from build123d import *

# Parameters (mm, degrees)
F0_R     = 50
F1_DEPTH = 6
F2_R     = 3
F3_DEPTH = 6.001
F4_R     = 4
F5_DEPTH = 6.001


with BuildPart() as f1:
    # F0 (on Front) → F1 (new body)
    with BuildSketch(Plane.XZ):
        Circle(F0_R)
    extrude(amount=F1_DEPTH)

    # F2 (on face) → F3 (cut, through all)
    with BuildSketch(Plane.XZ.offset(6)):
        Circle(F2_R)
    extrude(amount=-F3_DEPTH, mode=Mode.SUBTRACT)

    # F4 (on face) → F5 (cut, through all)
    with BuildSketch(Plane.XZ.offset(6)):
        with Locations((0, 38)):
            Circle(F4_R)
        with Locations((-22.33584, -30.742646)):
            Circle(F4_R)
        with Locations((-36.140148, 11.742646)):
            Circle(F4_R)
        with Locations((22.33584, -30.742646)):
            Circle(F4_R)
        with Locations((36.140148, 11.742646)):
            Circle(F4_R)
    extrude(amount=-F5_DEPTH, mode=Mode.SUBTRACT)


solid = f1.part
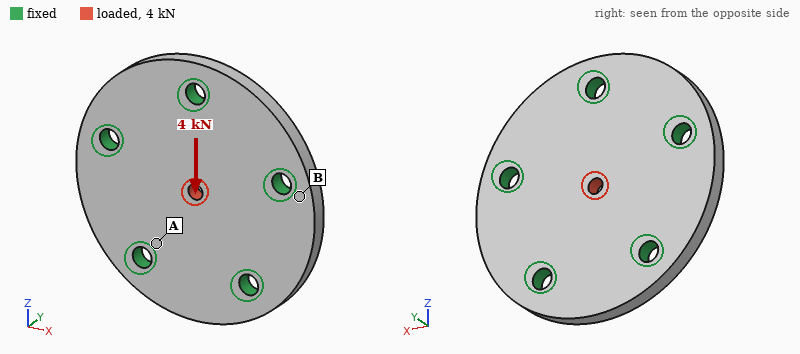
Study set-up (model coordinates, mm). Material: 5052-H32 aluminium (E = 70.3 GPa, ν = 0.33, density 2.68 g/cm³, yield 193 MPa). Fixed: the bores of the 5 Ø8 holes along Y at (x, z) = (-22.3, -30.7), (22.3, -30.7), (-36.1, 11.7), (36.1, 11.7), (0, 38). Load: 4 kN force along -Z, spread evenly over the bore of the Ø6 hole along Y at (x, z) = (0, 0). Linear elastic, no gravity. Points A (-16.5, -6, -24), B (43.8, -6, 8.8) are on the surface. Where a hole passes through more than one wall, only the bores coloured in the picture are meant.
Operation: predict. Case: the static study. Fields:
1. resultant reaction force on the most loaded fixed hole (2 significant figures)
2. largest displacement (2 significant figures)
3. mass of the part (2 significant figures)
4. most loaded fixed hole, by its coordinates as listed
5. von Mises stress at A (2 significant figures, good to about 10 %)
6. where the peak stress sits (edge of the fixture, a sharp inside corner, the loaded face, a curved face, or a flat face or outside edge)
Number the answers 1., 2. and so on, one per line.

1. 1.2 kN
2. 7.2 µm
3. 120 g
4. (0, 38)
5. 11 MPa
6. the loaded face
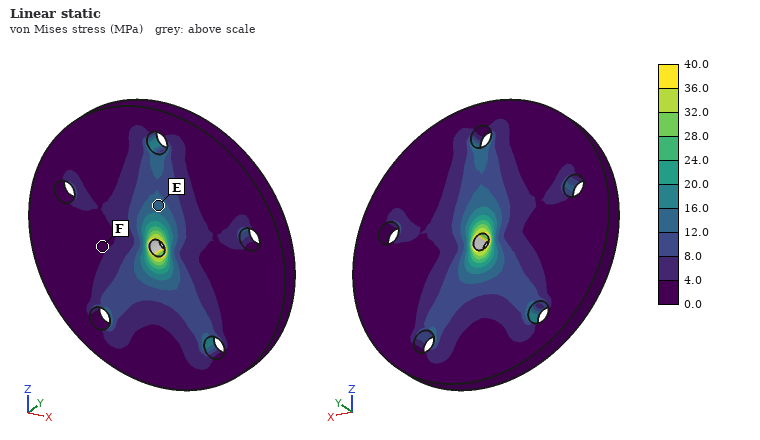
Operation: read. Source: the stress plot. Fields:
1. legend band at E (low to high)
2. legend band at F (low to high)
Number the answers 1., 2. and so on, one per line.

1. 12.0 to 16.0 MPa
2. 0.0 to 4.0 MPa
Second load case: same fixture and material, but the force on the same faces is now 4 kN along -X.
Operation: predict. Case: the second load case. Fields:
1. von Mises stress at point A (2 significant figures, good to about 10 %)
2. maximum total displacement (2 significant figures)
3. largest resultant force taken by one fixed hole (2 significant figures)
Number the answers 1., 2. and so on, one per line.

1. 7.9 MPa
2. 7.2 µm
3. 1.1 kN
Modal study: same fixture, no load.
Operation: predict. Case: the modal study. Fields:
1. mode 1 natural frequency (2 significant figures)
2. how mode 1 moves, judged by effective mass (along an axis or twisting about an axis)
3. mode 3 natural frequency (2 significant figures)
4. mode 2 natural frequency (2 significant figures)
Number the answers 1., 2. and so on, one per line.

1. 9100 Hz
2. along Y
3. 12 kHz
4. 12 kHz
